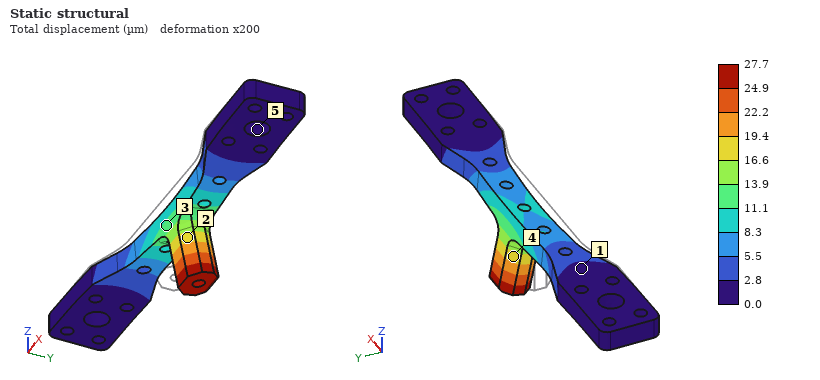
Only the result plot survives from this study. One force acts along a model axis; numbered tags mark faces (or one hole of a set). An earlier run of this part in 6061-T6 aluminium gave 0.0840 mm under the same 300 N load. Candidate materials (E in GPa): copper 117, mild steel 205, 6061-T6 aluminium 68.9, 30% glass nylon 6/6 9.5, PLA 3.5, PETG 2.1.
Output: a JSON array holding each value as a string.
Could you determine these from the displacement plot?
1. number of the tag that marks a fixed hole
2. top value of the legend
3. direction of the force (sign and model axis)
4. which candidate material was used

["5", "27.7 µm", "+Y", "mild steel"]
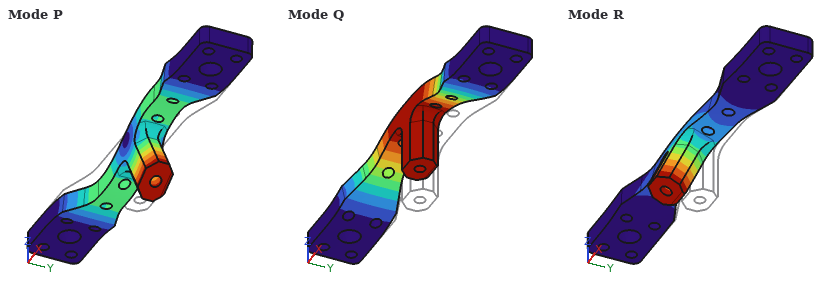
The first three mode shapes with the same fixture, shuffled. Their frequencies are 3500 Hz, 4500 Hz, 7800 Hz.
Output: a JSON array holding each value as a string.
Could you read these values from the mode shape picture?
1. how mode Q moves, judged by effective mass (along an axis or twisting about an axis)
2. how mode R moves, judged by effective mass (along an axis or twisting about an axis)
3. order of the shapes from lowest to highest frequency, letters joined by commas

["along Z", "along Y", "Q, R, P"]
